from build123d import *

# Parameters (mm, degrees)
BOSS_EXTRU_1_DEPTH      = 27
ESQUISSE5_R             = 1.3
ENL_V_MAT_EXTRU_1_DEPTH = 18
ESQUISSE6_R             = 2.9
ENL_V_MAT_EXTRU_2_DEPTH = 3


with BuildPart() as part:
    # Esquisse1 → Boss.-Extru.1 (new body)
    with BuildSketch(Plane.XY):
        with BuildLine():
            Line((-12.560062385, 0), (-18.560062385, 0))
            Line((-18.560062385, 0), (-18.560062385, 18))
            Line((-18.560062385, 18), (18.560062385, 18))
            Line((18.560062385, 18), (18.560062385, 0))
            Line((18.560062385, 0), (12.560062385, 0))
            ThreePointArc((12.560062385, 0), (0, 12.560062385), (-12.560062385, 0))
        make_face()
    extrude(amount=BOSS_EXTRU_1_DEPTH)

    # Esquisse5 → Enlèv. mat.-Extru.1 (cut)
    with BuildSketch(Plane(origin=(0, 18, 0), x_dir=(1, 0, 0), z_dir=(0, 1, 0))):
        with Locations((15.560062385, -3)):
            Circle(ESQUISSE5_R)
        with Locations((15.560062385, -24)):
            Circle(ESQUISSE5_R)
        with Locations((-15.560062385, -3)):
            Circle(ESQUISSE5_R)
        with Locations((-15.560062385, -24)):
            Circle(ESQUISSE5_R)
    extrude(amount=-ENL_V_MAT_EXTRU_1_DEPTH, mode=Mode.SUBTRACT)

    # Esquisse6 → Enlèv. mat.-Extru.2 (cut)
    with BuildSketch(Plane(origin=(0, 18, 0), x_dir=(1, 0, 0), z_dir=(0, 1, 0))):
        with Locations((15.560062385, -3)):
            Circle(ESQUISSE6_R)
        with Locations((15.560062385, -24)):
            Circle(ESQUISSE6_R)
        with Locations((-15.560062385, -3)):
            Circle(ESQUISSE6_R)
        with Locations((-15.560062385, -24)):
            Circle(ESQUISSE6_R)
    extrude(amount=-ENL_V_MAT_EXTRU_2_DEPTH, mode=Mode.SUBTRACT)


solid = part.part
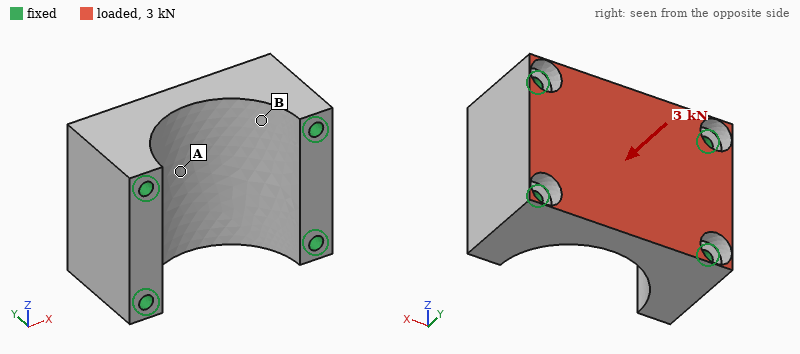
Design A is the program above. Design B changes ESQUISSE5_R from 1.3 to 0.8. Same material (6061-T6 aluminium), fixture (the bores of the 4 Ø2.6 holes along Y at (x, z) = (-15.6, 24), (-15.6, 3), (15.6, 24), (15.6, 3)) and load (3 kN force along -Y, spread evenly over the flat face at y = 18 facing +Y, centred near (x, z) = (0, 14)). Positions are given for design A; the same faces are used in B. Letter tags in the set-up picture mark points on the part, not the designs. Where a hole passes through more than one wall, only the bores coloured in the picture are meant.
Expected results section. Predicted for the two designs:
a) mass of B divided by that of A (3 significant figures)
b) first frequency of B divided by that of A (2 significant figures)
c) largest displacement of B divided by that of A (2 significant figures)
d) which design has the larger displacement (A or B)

1.02
0.94
1.1
B
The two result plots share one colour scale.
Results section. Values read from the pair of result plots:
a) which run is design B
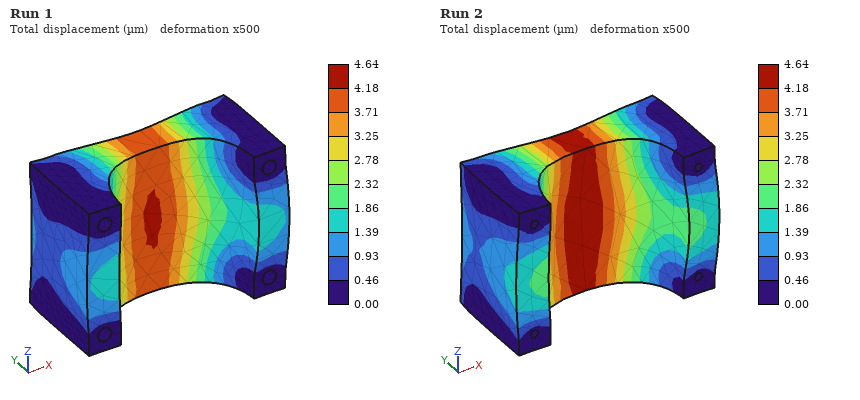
Run 2
